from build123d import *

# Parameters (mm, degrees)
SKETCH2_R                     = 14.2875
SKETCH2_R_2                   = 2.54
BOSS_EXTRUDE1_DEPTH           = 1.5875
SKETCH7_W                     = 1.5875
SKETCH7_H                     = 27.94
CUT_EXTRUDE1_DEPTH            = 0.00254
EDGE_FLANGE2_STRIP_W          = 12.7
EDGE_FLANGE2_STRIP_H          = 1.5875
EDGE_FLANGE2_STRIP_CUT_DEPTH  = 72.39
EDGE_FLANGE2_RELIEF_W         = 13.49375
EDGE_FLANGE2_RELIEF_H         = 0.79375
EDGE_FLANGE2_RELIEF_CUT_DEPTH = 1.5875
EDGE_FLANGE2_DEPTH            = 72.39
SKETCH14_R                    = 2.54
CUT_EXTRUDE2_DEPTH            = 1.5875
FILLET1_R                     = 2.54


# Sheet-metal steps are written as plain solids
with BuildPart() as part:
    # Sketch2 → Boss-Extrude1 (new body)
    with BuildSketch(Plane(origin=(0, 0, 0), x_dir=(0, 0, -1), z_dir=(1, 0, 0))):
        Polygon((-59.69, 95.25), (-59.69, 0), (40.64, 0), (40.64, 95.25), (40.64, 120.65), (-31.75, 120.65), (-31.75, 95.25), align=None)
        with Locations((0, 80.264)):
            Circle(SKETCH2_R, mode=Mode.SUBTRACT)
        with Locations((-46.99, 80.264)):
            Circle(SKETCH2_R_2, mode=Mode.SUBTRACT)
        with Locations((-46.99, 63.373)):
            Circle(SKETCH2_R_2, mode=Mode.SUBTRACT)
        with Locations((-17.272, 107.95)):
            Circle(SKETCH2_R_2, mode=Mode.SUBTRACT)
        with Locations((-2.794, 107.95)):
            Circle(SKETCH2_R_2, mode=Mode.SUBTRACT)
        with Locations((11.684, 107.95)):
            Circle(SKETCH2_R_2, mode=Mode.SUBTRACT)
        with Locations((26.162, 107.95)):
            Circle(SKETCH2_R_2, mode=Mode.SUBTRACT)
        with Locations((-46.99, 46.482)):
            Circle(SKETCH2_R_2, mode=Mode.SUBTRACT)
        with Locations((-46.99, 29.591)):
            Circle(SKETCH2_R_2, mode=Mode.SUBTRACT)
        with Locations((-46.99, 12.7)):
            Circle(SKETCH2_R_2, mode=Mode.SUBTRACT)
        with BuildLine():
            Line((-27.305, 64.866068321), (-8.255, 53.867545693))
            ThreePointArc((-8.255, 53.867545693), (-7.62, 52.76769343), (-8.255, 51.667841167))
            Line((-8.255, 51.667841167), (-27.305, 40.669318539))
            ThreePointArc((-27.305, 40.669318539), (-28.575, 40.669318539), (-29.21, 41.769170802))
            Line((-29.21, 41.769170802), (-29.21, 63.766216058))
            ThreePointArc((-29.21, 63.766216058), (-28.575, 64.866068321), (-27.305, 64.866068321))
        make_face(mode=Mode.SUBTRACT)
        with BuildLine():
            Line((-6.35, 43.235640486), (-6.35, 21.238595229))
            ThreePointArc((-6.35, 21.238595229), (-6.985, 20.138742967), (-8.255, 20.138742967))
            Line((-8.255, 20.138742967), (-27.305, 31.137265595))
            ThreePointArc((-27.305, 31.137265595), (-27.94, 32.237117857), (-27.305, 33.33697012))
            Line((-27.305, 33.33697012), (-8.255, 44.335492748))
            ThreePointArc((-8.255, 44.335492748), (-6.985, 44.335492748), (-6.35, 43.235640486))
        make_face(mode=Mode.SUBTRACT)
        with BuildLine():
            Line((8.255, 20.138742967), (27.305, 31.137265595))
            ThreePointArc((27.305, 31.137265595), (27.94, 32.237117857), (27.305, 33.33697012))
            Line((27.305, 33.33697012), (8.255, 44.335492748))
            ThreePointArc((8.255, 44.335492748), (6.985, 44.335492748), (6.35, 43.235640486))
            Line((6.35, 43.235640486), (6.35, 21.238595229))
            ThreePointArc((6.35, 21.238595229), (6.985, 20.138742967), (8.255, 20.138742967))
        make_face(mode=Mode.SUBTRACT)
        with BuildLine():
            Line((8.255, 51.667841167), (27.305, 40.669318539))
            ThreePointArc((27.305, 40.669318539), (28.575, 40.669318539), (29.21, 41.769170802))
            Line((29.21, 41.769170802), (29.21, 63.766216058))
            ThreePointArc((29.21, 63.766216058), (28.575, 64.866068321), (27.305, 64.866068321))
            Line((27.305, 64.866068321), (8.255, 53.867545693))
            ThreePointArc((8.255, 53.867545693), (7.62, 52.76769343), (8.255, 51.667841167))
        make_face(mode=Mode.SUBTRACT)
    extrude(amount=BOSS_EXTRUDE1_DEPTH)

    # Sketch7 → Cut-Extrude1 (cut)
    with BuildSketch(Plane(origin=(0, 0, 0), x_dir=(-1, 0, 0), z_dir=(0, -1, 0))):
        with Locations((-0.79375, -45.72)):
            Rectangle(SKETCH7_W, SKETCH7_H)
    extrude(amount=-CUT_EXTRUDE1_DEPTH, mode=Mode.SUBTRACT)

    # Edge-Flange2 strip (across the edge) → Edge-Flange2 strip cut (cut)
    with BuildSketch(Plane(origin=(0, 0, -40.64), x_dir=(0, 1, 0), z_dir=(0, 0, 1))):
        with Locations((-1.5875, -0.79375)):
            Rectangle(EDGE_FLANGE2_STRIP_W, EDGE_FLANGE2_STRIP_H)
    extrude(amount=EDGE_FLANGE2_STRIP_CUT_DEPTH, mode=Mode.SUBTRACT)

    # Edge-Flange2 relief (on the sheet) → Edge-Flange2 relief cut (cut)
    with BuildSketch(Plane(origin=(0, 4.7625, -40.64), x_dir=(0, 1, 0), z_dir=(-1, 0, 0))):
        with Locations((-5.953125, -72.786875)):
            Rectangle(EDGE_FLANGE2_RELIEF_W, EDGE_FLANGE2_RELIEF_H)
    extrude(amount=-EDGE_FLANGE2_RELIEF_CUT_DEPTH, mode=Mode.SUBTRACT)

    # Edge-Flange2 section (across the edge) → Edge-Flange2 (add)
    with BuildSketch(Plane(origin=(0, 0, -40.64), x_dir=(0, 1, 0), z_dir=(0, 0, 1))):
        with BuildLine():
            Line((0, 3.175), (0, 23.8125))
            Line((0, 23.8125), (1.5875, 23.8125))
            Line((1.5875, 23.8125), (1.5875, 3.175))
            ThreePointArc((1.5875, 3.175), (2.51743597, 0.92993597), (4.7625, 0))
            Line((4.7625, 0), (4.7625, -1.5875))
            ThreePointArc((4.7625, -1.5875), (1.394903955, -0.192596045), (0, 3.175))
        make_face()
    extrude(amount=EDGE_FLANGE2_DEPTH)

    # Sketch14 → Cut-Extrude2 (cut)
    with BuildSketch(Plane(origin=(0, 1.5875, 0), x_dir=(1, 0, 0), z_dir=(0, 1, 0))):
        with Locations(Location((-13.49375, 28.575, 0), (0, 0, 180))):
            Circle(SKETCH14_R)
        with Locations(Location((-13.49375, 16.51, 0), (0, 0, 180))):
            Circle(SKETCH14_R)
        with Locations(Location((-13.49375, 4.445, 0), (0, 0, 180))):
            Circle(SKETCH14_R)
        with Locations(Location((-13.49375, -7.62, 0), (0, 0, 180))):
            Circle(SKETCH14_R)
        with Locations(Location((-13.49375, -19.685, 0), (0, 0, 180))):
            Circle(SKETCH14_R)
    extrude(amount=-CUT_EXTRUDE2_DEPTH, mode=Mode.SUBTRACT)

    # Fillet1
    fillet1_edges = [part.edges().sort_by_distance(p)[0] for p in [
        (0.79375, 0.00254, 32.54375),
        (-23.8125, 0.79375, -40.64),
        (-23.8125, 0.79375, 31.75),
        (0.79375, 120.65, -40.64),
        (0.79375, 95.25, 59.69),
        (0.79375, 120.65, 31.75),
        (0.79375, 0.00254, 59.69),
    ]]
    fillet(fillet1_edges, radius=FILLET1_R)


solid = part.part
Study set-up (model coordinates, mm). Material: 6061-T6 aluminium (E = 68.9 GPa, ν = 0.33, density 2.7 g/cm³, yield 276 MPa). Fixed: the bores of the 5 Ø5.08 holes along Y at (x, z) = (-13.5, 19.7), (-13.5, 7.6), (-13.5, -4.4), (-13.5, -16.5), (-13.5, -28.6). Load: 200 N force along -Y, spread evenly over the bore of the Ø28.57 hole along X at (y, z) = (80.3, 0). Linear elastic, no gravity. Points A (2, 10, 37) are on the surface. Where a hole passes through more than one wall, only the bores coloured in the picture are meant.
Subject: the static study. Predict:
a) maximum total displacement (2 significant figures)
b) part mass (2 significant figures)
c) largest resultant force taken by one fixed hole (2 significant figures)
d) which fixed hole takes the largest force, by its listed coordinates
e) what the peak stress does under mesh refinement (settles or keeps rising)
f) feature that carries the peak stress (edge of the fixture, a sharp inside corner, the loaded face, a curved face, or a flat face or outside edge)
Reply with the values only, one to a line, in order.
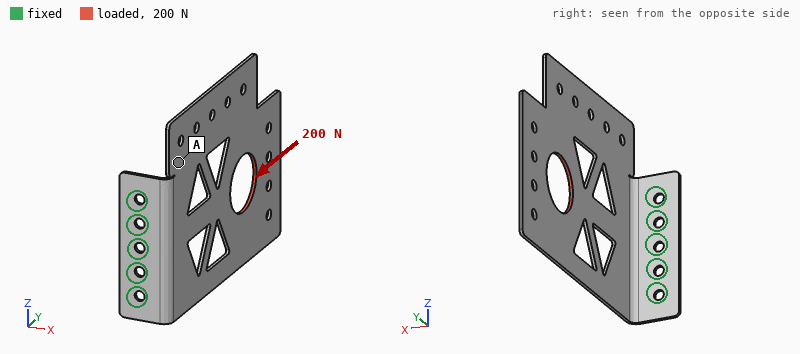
1.2 mm
47 g
60 N
(-13.5, 19.7)
keeps rising
edge of the fixture
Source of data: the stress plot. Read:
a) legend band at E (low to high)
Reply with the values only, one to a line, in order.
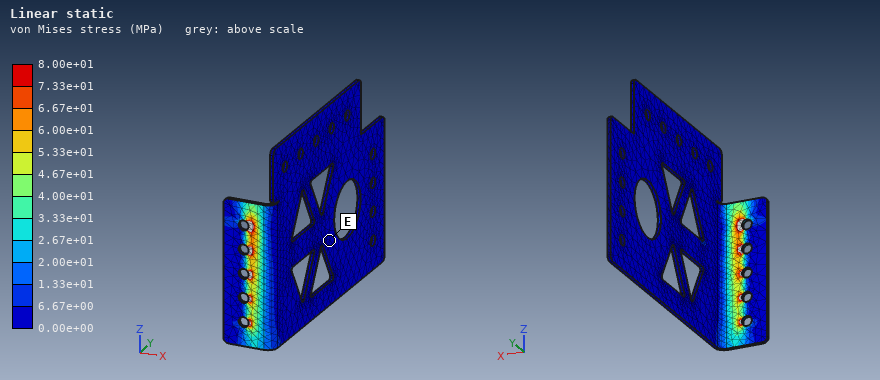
0.00e+00 to 6.67e+00 MPa
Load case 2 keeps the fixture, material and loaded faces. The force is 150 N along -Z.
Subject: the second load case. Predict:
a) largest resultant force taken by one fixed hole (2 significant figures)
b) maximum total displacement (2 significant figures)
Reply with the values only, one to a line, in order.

200 N
1.4 mm
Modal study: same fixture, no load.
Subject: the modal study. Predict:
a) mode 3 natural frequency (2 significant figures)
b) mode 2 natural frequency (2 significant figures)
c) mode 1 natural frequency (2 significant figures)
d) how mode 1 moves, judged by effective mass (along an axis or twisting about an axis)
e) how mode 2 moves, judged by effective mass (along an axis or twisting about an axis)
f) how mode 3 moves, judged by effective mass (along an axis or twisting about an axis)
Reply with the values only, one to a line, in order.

440 Hz
210 Hz
75 Hz
along X
twisting about Y
along Z
